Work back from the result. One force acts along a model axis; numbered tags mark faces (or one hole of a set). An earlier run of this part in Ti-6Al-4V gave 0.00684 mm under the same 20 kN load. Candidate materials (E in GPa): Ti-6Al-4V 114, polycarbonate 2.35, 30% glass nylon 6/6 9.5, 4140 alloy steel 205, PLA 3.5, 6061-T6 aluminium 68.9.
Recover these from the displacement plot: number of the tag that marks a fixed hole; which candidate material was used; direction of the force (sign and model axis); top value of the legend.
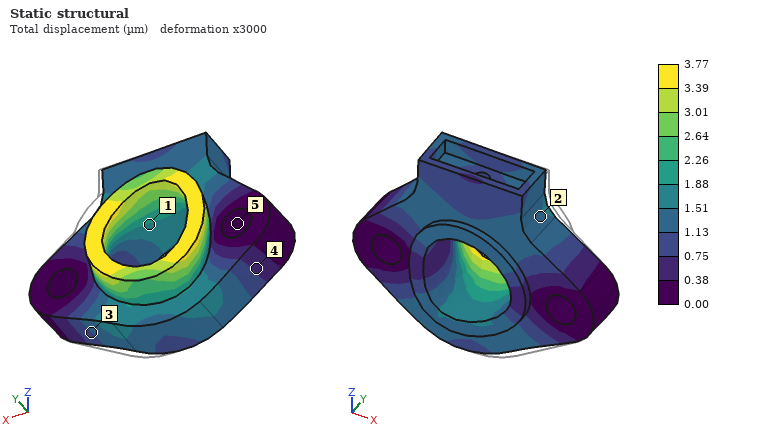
5
4140 alloy steel
-X
3.77 µm
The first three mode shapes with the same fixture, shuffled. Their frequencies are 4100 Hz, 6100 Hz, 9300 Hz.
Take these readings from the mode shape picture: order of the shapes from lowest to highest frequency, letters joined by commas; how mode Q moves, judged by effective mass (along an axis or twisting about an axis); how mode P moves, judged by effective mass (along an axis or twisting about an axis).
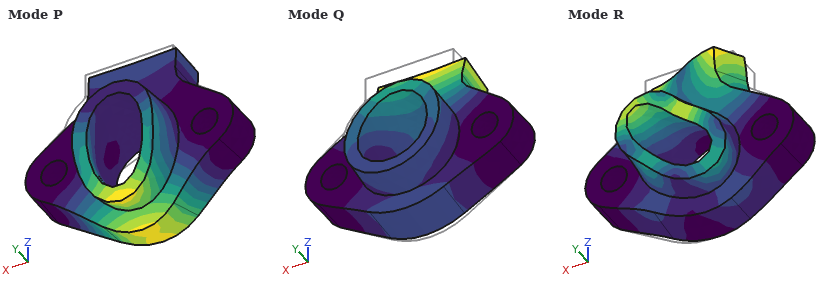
Q, P, R
along Y
along Y
